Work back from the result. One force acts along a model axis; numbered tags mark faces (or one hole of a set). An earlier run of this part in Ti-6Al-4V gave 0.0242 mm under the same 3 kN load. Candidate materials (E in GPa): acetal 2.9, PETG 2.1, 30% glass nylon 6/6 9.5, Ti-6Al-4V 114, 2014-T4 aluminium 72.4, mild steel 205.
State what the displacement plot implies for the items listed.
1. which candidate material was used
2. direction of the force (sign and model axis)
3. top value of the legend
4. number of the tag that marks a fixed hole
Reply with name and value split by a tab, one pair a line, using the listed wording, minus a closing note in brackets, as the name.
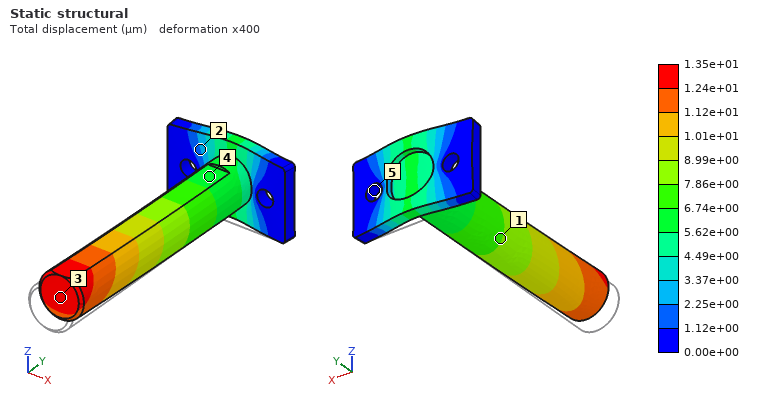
which candidate material was used	mild steel
direction of the force	+Y
top value of the legend	1.35e+01 µm
number of the tag that marks a fixed hole	5
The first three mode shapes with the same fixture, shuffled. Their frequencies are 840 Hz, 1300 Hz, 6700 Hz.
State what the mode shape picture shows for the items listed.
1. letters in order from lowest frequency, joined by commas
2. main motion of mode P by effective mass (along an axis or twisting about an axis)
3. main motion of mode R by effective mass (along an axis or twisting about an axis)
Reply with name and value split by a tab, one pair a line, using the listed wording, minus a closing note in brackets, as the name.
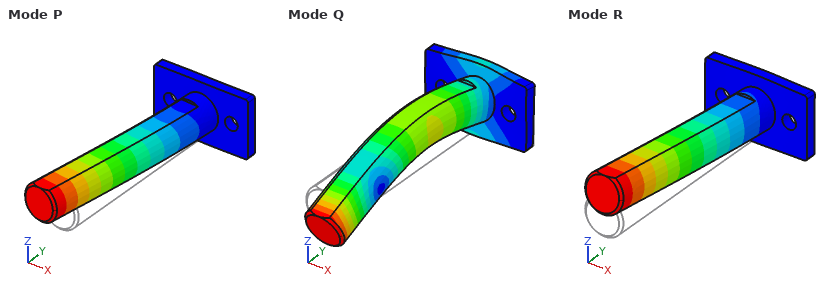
letters in order from lowest frequency, joined by commas	R, P, Q
main motion of mode P by effective mass	along X
main motion of mode R by effective mass	along Z
